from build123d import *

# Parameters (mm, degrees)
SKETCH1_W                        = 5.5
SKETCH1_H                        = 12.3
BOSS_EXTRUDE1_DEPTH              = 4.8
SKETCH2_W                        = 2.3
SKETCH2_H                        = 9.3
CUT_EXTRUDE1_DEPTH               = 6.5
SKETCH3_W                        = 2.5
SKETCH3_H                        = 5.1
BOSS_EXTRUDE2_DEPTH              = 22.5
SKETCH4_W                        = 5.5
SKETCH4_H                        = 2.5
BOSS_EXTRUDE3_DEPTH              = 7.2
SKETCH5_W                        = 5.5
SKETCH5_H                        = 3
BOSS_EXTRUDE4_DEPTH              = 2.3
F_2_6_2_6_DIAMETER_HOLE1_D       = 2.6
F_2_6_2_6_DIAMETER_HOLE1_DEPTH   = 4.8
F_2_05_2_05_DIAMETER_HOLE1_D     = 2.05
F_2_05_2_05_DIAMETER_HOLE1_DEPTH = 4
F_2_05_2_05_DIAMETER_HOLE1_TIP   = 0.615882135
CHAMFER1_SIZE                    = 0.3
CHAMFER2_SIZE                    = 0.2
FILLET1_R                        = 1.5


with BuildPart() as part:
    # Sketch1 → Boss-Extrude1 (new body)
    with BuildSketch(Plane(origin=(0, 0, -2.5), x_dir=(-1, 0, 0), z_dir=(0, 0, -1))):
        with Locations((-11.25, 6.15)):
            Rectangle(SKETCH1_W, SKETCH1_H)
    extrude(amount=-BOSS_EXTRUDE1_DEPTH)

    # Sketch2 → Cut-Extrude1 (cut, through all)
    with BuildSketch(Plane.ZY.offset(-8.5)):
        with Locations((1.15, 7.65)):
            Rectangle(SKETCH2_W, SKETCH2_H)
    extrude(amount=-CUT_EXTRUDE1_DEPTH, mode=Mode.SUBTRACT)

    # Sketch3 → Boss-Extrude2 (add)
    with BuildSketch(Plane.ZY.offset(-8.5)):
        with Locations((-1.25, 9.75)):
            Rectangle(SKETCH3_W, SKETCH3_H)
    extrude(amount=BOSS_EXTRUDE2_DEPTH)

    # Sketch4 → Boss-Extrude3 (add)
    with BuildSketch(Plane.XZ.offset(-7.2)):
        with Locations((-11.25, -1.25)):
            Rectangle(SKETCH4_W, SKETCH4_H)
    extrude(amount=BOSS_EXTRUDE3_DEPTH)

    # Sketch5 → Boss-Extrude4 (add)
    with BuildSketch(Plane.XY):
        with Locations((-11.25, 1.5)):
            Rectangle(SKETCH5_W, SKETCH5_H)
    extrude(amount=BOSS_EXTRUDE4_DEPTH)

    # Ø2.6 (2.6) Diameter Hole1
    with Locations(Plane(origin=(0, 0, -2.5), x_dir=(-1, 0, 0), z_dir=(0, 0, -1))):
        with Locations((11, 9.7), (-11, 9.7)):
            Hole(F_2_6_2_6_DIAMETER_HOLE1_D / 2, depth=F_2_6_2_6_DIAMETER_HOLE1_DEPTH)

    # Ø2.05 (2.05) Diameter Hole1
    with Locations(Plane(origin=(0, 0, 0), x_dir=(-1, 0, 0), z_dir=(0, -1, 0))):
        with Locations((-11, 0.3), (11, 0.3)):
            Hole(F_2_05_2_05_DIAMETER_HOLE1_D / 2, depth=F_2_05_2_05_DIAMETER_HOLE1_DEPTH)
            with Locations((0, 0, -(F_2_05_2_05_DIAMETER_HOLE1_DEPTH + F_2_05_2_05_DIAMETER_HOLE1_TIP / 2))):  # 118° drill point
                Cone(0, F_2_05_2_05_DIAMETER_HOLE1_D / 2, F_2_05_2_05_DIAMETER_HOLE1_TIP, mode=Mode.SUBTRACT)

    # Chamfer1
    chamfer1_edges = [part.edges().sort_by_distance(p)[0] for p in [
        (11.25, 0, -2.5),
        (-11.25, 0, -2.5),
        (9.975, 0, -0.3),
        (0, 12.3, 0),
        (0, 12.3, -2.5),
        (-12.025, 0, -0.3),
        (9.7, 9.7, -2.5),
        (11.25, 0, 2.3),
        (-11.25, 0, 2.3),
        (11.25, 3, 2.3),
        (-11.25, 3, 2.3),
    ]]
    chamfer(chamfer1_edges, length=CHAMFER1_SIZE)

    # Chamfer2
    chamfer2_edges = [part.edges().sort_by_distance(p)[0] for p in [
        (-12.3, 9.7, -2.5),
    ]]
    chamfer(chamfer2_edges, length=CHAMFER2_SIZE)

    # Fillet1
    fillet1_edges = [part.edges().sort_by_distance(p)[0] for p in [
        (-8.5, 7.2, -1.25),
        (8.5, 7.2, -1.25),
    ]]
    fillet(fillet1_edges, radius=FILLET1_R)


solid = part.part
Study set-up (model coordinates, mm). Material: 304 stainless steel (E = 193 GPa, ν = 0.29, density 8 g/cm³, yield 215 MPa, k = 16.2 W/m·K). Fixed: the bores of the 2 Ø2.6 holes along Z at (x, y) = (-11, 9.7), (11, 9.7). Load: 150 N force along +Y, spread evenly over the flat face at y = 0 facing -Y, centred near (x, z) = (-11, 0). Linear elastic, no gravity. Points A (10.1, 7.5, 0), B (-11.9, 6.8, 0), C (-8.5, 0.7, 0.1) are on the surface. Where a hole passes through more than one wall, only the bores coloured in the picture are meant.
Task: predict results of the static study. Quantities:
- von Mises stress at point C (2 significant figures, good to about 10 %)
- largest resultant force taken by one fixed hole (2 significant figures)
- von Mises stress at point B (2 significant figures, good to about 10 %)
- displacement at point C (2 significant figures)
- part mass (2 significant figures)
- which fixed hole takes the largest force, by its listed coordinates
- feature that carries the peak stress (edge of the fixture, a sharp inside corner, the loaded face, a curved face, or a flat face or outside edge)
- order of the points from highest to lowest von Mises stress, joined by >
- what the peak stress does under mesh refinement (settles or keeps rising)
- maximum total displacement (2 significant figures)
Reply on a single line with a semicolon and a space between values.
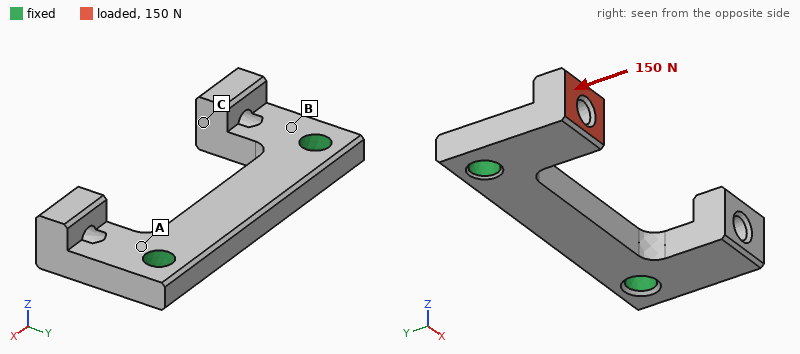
15 MPa; 150 N; 41 MPa; 4.9 µm; 4.6 g; (-11, 9.7); a sharp inside corner; B > C > A; keeps rising; 6.8 µm
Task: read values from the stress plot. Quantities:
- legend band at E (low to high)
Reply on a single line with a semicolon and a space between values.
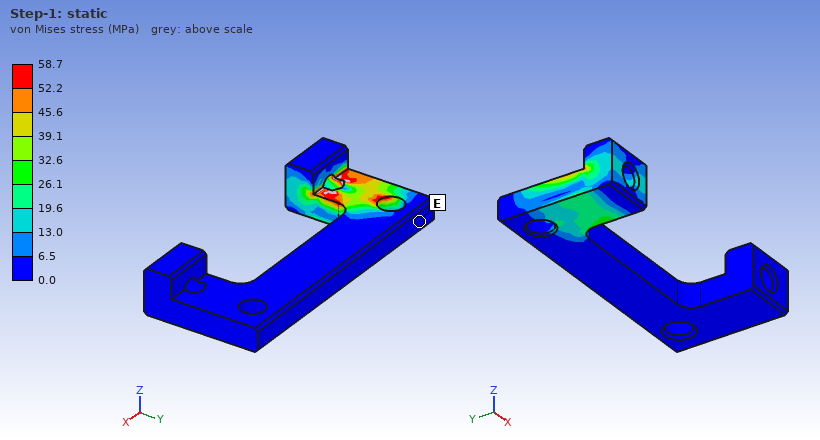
0.0 to 6.5 MPa
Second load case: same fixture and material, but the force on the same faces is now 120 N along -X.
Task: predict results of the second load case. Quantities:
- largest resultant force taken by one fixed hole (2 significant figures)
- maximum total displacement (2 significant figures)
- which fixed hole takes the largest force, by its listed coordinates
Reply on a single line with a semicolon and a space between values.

100 N; 9.3 µm; (-11, 9.7)
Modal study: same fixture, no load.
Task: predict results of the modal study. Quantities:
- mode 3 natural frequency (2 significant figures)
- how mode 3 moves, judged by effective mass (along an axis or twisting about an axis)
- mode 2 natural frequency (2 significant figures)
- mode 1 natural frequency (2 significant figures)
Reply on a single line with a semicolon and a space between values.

27 kHz; along Z; 19 kHz; 18 kHz
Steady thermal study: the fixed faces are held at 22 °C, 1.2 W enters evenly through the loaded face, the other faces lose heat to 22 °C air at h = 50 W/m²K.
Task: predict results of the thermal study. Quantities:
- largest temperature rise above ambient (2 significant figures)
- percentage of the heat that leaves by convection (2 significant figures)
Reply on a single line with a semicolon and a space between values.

43 K; 21 %
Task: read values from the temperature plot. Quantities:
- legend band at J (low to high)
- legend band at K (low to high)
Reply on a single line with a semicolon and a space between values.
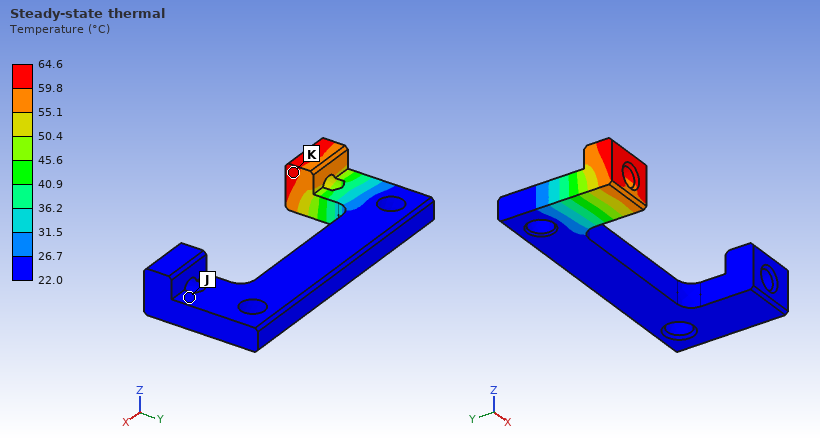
22.0 to 26.7 °C; 59.8 to 64.6 °C
